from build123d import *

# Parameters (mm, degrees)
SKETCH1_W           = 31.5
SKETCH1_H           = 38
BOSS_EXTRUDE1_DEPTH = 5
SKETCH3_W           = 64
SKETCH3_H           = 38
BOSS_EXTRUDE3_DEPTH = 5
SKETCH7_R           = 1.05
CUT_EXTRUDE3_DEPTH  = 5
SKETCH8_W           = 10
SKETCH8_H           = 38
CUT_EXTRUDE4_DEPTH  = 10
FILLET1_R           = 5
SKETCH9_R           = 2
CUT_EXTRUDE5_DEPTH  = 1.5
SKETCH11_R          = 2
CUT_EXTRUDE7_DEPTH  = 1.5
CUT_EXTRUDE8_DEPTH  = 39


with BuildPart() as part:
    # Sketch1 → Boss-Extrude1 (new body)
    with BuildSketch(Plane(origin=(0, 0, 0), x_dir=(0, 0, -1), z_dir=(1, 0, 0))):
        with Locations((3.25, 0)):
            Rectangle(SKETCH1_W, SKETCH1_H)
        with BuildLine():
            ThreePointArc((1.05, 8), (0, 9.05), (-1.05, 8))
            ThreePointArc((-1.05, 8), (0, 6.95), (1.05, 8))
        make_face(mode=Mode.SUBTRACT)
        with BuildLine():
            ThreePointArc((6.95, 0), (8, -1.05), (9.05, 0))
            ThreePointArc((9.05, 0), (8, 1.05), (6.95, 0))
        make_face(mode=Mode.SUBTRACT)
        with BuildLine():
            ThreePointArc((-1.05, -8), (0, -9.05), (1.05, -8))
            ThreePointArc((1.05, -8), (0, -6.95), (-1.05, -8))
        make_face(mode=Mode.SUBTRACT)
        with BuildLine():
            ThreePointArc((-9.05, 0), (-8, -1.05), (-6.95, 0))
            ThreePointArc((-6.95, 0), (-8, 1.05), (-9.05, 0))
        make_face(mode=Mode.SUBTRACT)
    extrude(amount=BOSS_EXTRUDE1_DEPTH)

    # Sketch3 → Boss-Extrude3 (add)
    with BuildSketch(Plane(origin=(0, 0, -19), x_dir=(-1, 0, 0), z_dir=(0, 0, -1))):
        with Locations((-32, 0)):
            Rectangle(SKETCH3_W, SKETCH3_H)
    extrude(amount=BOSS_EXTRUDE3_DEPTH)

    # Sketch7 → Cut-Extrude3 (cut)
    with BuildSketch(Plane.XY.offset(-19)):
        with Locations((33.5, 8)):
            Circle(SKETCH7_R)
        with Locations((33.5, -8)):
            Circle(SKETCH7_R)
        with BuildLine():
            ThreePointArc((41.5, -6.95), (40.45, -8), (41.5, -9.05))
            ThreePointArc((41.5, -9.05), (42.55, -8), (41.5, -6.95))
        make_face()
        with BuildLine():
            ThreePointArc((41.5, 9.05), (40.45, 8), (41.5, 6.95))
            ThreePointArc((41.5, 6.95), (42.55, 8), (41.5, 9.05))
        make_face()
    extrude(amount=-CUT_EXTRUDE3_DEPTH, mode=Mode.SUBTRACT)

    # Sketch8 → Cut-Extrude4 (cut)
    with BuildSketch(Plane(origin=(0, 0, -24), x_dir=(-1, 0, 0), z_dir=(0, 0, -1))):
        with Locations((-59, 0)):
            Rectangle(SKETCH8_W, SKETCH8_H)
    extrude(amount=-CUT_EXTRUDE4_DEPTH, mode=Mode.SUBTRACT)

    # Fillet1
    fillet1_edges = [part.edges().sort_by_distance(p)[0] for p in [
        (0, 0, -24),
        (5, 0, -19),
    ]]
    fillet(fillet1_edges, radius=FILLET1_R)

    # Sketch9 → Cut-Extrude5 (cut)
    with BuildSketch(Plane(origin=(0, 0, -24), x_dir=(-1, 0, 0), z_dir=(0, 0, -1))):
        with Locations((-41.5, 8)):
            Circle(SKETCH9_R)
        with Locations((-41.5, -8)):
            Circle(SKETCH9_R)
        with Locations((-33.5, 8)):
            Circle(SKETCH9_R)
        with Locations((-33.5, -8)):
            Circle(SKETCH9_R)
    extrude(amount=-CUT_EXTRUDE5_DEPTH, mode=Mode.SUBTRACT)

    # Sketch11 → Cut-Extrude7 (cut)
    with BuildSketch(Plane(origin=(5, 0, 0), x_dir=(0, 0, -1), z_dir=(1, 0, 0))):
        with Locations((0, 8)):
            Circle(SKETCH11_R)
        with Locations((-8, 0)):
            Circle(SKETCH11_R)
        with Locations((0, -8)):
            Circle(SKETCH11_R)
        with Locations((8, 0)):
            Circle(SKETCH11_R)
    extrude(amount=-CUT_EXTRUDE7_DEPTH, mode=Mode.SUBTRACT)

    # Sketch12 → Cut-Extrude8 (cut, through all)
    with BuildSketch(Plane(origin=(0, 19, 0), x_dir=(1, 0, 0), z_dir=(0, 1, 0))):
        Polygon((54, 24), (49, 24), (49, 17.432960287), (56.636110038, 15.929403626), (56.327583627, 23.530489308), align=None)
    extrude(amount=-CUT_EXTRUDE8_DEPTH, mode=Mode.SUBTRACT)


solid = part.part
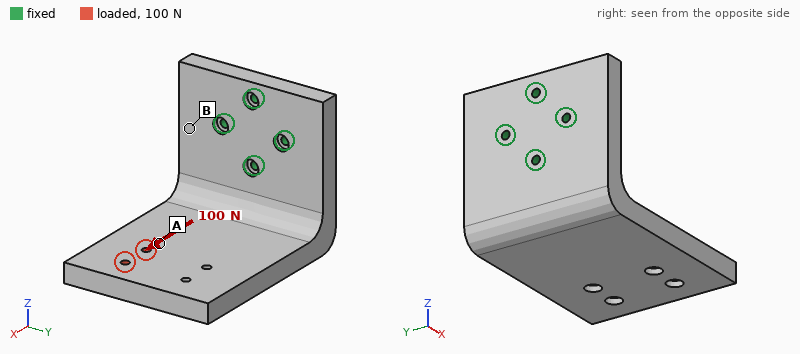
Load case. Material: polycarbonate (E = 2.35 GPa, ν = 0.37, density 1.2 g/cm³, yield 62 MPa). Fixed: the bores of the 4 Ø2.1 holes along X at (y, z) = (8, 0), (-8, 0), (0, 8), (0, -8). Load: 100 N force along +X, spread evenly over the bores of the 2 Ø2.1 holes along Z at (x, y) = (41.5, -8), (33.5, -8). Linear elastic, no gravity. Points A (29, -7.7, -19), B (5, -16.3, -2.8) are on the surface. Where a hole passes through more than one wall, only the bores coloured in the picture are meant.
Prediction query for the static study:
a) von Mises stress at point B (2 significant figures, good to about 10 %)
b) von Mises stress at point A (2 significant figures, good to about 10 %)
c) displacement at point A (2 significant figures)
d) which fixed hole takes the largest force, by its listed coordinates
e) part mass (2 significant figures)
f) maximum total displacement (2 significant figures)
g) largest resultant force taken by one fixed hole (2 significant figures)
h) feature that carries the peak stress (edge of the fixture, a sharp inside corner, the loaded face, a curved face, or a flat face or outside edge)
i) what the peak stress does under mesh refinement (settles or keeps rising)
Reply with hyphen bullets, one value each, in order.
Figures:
- 5.2 MPa
- 2.0 MPa
- 0.50 mm
- (0, -8)
- 18 g
- 0.85 mm
- 170 N
- edge of the fixture
- keeps rising
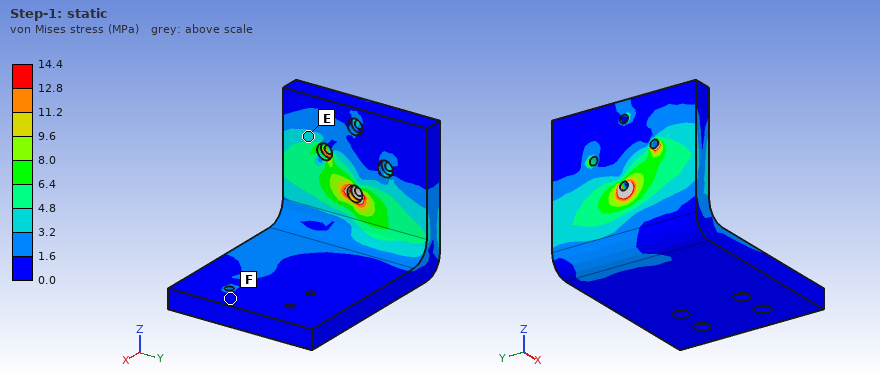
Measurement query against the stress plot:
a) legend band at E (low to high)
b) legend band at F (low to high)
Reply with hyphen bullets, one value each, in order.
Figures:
- 3.2 to 4.8 MPa
- 0.0 to 1.6 MPa
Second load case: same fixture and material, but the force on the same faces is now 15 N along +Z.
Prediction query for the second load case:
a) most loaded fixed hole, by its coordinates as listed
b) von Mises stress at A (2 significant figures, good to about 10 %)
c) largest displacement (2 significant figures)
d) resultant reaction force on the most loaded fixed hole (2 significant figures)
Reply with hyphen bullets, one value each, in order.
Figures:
- (0, -8)
- 1.1 MPa
- 0.68 mm
- 40 N
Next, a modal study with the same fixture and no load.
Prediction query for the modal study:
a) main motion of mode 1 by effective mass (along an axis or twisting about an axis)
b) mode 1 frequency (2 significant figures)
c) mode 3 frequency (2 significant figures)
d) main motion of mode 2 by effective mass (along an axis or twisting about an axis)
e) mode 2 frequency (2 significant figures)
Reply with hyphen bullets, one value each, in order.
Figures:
- along Z
- 370 Hz
- 1400 Hz
- along Y
- 550 Hz
